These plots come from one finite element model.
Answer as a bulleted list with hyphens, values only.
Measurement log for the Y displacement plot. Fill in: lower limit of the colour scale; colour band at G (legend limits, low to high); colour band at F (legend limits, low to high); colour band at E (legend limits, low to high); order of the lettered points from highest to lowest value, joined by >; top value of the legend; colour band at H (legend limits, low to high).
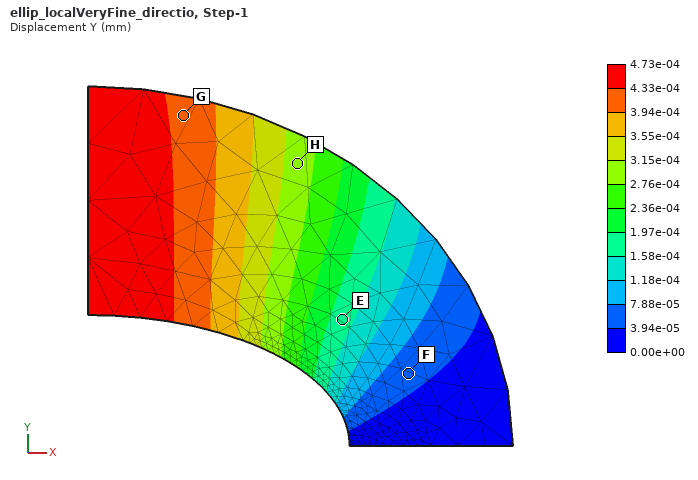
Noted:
- 0.00e+00 mm
- 3.94e-04 to 4.33e-04 mm
- 3.94e-05 to 7.88e-05 mm
- 1.58e-04 to 1.97e-04 mm
- G > H > E > F
- 4.73e-04 mm
- 2.76e-04 to 3.15e-04 mm
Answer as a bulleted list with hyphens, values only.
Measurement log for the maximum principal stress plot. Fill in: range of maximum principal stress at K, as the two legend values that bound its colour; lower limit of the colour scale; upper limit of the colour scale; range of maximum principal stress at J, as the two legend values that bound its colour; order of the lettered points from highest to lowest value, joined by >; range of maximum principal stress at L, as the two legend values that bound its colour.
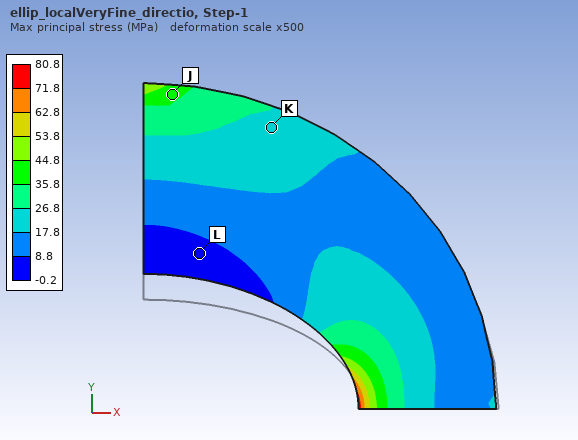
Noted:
- 17.8 to 26.8 MPa
- -0.2 MPa
- 80.8 MPa
- 35.8 to 44.8 MPa
- J > K > L
- -0.2 to 8.8 MPa
